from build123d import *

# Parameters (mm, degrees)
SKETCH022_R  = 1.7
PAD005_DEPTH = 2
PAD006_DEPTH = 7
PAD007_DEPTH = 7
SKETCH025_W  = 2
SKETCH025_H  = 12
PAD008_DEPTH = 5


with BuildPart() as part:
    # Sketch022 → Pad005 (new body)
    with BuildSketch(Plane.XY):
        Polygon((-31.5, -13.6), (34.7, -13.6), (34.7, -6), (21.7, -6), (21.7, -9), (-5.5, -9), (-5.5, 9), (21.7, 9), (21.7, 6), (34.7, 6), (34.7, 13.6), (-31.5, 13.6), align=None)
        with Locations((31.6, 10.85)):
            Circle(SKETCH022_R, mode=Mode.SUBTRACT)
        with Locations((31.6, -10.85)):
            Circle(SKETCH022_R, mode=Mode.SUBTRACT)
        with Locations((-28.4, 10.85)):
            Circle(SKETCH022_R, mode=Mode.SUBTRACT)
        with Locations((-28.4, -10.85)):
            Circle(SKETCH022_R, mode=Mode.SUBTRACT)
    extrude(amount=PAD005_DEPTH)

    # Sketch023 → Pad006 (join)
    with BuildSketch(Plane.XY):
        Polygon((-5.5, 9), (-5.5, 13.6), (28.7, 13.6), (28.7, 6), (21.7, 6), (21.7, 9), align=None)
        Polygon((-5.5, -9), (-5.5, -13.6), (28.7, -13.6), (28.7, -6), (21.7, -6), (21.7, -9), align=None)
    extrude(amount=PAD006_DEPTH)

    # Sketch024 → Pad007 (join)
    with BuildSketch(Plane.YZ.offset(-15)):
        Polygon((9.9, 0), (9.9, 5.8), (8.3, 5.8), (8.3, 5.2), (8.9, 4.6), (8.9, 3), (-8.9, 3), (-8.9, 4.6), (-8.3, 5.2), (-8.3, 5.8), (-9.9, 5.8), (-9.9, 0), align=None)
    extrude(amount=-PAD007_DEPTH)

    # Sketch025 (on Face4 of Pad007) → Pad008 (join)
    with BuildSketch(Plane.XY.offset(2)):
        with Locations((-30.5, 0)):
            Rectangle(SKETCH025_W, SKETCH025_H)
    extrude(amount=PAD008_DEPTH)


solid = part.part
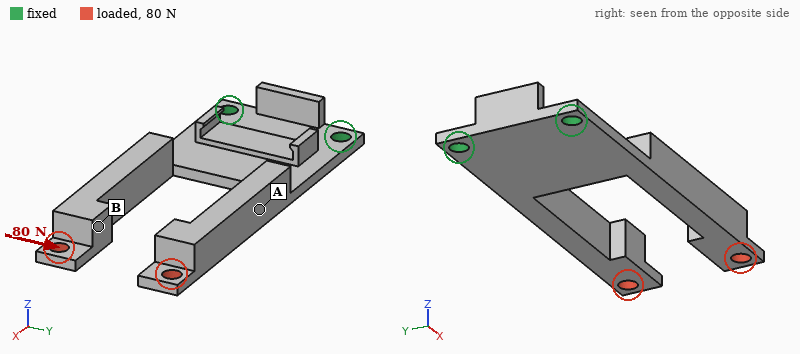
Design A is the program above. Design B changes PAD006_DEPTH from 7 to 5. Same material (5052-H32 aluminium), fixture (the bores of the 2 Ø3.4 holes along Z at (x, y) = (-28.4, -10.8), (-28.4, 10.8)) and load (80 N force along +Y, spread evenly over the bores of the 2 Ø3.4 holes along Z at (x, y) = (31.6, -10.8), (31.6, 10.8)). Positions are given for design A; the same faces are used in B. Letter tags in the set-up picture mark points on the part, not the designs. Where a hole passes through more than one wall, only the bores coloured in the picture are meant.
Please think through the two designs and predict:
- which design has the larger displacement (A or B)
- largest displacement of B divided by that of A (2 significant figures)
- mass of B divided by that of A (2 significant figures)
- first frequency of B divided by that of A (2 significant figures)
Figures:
B
1.1
0.84
1.1
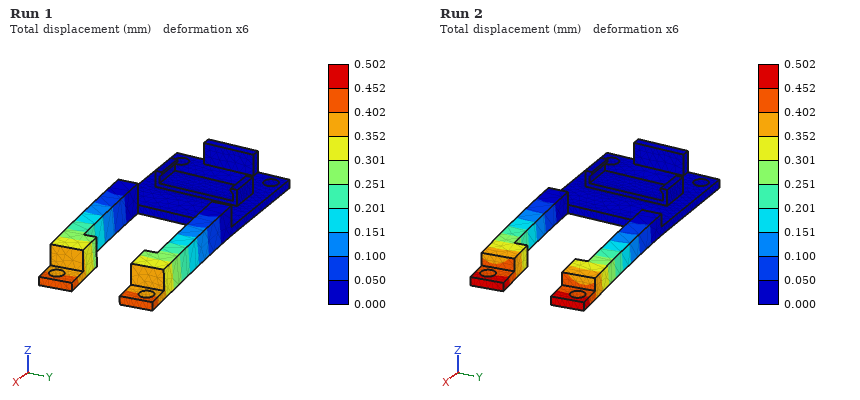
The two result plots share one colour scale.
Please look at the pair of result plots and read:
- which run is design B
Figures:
Run 2
